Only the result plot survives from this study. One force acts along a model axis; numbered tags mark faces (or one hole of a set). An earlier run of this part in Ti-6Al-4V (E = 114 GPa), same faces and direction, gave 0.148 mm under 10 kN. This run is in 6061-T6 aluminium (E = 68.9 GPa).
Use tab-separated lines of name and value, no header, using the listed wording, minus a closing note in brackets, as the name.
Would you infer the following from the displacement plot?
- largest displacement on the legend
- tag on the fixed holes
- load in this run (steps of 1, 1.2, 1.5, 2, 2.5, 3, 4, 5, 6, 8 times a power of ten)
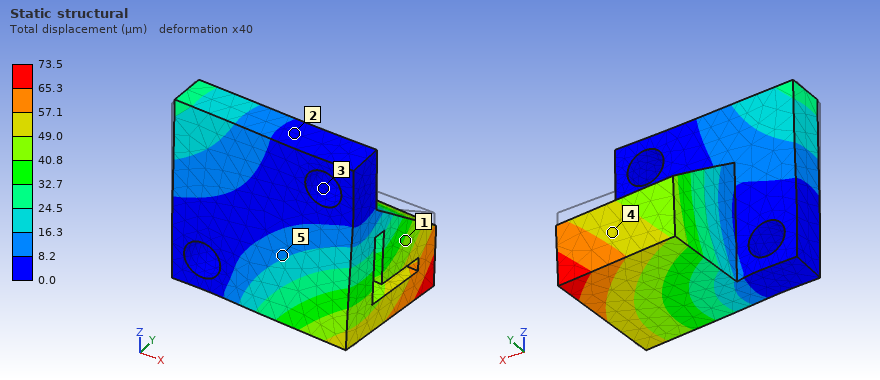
largest displacement on the legend	73.5 µm
tag on the fixed holes	3
load in this run	3 kN
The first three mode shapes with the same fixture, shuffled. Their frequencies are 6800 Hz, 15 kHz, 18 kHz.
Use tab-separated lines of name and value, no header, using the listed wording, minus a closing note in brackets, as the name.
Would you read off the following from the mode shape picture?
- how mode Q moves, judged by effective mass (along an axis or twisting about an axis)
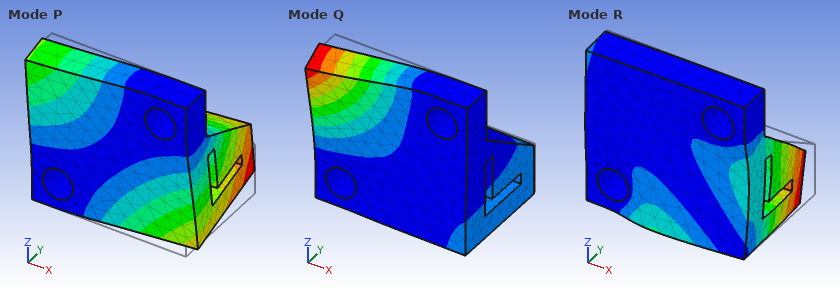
how mode Q moves, judged by effective mass	along Y
